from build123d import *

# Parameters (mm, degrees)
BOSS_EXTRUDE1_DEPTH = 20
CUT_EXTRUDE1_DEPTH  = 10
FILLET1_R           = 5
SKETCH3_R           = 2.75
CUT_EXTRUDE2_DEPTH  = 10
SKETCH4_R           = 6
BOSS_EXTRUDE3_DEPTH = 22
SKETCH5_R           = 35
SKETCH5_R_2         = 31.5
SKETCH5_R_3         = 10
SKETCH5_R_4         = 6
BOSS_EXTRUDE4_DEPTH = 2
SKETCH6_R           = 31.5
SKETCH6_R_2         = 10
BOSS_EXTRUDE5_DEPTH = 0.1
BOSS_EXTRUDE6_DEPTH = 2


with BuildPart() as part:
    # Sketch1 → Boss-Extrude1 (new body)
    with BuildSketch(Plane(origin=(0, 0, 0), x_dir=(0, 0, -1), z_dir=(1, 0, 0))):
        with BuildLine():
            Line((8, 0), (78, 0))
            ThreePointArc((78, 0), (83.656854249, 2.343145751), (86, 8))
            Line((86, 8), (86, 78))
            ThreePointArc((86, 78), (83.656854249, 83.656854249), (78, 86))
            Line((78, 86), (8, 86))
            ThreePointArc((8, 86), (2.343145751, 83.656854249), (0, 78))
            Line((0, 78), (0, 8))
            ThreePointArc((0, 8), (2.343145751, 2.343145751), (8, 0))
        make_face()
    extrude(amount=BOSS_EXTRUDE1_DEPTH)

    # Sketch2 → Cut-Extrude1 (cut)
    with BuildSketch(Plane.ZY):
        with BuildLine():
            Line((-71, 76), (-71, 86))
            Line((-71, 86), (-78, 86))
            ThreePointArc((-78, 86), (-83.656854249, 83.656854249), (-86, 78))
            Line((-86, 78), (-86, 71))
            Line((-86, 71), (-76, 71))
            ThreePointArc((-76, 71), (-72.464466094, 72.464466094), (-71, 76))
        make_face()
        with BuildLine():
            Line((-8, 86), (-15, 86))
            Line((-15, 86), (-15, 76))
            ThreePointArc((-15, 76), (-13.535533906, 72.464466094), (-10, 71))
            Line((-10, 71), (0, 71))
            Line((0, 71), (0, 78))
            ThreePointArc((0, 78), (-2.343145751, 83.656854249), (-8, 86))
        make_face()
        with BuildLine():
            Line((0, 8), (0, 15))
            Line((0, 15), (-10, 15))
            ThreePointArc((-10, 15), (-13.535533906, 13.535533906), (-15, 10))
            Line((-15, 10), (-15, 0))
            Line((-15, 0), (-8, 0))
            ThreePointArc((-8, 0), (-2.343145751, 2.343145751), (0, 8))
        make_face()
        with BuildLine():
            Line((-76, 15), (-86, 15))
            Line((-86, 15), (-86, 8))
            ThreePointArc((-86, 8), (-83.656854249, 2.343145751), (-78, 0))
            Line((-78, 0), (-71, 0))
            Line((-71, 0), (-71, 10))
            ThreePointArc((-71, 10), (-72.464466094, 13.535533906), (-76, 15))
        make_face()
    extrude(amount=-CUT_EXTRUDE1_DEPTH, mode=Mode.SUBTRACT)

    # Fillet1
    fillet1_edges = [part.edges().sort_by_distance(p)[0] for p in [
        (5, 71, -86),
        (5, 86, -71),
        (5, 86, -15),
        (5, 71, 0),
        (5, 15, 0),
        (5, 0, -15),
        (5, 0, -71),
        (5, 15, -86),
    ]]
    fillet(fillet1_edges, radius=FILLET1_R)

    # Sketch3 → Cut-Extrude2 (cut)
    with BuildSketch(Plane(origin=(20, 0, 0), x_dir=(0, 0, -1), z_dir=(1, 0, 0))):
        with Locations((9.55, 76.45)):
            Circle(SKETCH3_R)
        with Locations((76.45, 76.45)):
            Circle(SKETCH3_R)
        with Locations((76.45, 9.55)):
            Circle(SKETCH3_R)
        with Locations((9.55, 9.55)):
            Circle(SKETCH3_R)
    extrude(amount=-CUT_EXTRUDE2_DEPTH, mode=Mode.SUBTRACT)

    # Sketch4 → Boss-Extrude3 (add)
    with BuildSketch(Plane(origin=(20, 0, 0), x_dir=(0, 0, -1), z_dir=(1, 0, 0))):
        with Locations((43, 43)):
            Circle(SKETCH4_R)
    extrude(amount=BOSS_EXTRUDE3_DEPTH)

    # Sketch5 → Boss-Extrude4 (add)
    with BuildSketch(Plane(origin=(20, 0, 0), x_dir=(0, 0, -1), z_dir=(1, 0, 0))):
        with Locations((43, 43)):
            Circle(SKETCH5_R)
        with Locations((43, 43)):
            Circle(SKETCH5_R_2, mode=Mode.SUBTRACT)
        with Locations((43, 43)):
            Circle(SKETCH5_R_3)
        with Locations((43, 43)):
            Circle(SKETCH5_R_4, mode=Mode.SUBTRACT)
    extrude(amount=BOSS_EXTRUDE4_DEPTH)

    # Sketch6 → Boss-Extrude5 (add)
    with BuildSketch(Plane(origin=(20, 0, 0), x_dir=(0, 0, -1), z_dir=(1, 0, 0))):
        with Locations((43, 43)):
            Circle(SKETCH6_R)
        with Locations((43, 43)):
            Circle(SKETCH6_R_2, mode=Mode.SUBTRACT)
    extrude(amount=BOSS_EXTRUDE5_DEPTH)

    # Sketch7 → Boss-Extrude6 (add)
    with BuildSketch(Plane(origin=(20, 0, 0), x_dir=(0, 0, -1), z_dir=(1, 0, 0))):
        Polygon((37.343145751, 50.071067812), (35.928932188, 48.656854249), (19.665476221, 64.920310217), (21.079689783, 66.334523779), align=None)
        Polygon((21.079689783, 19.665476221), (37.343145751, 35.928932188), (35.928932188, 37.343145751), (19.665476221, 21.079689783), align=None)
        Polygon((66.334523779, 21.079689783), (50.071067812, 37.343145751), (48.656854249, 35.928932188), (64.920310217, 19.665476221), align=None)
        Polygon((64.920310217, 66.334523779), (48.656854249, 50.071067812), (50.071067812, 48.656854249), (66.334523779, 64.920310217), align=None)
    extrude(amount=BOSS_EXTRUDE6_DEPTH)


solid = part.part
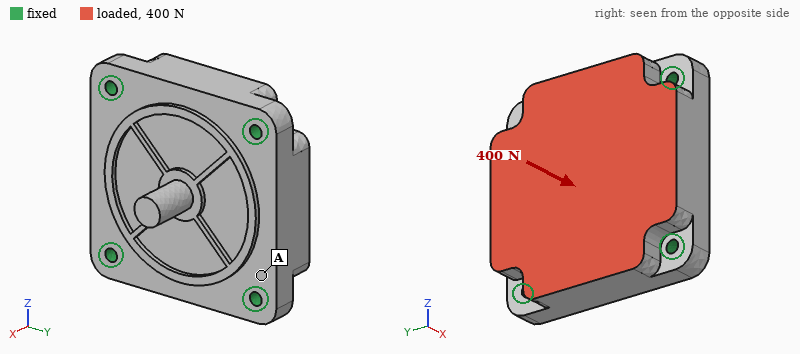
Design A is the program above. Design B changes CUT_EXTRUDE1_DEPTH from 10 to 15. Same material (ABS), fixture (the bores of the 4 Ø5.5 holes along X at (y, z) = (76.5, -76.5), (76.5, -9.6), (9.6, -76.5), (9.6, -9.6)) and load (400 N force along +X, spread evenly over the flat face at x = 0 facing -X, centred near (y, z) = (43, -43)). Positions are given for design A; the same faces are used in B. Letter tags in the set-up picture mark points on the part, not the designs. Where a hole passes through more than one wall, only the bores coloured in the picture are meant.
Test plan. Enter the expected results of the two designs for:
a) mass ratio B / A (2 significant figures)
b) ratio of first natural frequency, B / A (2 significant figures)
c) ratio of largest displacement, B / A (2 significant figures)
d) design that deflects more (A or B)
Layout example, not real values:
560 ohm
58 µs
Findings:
0.97
0.83
1.4
B
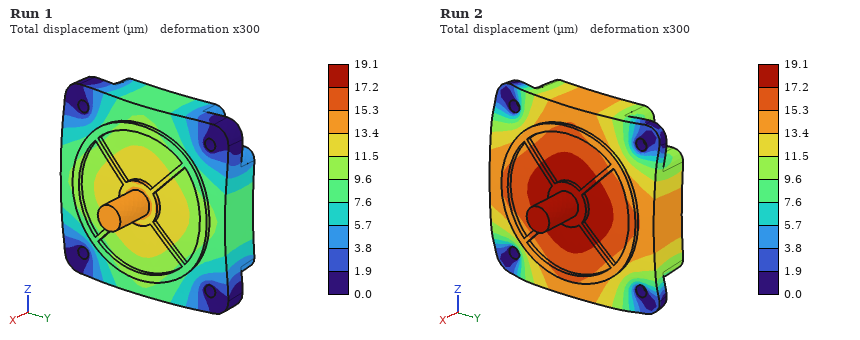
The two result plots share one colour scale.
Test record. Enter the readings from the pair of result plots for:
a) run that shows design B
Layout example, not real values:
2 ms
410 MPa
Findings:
Run 2
